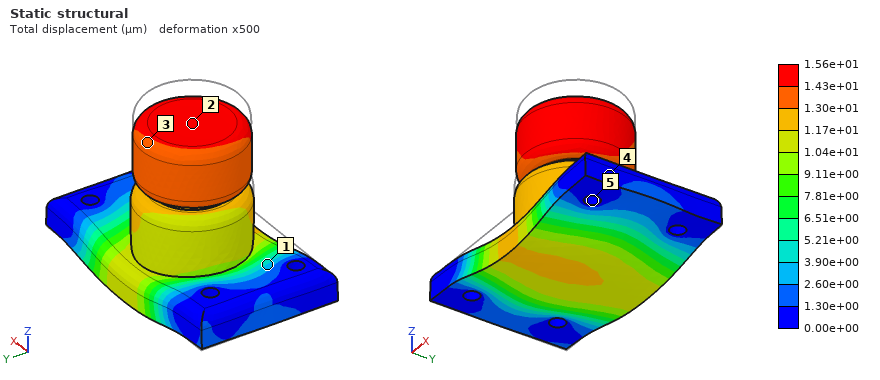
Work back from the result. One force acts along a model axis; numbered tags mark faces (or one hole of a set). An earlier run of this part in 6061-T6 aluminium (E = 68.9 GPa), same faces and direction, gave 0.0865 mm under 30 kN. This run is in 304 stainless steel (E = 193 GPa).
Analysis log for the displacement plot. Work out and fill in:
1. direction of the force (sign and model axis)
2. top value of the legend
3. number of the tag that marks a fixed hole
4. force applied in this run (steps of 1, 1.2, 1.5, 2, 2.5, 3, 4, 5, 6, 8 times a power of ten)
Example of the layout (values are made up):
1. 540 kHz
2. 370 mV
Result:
1. -Z
2. 1.56e+01 µm
3. 5
4. 15 kN
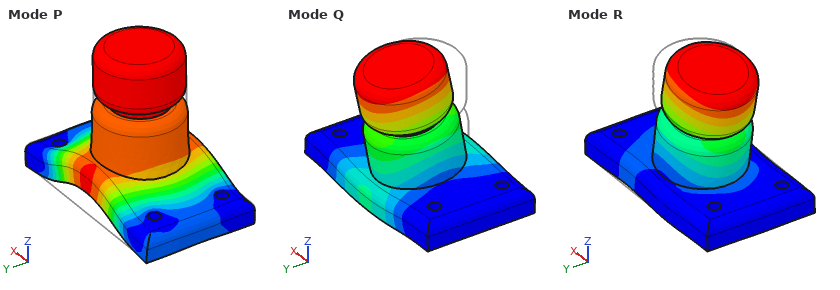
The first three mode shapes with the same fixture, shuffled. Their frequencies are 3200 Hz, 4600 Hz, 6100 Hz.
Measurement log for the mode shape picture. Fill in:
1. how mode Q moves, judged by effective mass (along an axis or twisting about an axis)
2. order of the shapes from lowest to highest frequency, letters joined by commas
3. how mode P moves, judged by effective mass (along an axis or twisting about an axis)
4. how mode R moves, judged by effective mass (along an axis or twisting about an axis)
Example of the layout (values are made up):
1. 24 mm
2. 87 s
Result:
1. along Y
2. Q, R, P
3. along Z
4. along X
